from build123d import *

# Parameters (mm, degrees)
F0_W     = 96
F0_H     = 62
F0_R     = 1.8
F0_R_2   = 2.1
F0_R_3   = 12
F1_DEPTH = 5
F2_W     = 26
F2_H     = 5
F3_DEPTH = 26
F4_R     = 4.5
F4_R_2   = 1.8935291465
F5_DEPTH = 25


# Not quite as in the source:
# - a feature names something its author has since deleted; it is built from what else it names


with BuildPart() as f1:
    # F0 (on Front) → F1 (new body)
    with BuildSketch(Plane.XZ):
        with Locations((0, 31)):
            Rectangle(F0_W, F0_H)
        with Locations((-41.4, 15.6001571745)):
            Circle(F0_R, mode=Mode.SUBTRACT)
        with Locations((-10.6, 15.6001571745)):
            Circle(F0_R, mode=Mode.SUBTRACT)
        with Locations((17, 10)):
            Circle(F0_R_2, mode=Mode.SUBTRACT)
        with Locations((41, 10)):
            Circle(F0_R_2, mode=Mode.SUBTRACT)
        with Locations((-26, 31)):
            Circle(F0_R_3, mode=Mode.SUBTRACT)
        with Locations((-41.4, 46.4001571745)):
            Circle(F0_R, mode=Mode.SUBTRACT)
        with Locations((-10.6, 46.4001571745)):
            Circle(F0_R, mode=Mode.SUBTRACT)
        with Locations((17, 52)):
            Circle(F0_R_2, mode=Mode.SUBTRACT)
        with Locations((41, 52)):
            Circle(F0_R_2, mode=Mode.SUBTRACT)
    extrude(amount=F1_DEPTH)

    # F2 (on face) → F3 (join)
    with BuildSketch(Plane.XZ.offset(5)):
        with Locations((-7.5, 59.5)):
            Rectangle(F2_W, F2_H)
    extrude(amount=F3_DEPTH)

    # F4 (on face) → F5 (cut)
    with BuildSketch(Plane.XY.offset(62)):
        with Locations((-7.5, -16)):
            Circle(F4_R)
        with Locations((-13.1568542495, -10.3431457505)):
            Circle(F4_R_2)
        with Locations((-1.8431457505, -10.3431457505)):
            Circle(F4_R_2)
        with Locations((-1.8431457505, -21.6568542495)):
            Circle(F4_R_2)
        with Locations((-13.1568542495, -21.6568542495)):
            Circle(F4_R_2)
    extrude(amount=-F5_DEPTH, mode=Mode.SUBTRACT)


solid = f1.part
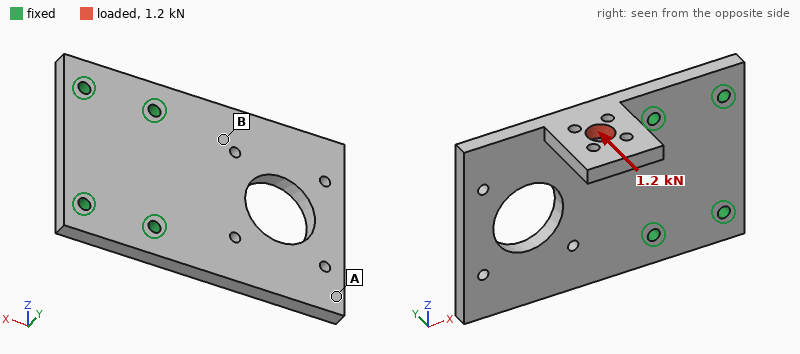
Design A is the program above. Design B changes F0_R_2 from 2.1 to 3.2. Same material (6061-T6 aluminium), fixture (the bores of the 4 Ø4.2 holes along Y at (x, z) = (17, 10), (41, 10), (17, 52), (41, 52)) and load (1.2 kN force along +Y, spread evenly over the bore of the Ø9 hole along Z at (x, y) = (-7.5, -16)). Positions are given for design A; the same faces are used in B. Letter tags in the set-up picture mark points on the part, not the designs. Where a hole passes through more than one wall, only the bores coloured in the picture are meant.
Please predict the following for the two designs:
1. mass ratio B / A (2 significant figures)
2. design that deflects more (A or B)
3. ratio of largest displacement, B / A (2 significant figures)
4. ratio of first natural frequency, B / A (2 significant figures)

0.99
A
0.89
1.1
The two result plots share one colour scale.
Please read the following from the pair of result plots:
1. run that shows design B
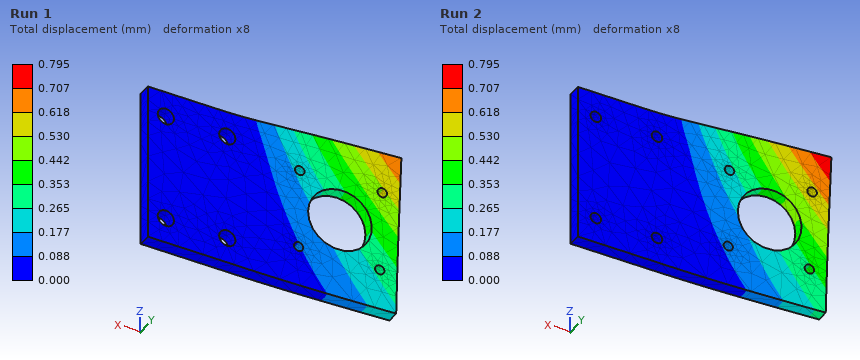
Run 1
